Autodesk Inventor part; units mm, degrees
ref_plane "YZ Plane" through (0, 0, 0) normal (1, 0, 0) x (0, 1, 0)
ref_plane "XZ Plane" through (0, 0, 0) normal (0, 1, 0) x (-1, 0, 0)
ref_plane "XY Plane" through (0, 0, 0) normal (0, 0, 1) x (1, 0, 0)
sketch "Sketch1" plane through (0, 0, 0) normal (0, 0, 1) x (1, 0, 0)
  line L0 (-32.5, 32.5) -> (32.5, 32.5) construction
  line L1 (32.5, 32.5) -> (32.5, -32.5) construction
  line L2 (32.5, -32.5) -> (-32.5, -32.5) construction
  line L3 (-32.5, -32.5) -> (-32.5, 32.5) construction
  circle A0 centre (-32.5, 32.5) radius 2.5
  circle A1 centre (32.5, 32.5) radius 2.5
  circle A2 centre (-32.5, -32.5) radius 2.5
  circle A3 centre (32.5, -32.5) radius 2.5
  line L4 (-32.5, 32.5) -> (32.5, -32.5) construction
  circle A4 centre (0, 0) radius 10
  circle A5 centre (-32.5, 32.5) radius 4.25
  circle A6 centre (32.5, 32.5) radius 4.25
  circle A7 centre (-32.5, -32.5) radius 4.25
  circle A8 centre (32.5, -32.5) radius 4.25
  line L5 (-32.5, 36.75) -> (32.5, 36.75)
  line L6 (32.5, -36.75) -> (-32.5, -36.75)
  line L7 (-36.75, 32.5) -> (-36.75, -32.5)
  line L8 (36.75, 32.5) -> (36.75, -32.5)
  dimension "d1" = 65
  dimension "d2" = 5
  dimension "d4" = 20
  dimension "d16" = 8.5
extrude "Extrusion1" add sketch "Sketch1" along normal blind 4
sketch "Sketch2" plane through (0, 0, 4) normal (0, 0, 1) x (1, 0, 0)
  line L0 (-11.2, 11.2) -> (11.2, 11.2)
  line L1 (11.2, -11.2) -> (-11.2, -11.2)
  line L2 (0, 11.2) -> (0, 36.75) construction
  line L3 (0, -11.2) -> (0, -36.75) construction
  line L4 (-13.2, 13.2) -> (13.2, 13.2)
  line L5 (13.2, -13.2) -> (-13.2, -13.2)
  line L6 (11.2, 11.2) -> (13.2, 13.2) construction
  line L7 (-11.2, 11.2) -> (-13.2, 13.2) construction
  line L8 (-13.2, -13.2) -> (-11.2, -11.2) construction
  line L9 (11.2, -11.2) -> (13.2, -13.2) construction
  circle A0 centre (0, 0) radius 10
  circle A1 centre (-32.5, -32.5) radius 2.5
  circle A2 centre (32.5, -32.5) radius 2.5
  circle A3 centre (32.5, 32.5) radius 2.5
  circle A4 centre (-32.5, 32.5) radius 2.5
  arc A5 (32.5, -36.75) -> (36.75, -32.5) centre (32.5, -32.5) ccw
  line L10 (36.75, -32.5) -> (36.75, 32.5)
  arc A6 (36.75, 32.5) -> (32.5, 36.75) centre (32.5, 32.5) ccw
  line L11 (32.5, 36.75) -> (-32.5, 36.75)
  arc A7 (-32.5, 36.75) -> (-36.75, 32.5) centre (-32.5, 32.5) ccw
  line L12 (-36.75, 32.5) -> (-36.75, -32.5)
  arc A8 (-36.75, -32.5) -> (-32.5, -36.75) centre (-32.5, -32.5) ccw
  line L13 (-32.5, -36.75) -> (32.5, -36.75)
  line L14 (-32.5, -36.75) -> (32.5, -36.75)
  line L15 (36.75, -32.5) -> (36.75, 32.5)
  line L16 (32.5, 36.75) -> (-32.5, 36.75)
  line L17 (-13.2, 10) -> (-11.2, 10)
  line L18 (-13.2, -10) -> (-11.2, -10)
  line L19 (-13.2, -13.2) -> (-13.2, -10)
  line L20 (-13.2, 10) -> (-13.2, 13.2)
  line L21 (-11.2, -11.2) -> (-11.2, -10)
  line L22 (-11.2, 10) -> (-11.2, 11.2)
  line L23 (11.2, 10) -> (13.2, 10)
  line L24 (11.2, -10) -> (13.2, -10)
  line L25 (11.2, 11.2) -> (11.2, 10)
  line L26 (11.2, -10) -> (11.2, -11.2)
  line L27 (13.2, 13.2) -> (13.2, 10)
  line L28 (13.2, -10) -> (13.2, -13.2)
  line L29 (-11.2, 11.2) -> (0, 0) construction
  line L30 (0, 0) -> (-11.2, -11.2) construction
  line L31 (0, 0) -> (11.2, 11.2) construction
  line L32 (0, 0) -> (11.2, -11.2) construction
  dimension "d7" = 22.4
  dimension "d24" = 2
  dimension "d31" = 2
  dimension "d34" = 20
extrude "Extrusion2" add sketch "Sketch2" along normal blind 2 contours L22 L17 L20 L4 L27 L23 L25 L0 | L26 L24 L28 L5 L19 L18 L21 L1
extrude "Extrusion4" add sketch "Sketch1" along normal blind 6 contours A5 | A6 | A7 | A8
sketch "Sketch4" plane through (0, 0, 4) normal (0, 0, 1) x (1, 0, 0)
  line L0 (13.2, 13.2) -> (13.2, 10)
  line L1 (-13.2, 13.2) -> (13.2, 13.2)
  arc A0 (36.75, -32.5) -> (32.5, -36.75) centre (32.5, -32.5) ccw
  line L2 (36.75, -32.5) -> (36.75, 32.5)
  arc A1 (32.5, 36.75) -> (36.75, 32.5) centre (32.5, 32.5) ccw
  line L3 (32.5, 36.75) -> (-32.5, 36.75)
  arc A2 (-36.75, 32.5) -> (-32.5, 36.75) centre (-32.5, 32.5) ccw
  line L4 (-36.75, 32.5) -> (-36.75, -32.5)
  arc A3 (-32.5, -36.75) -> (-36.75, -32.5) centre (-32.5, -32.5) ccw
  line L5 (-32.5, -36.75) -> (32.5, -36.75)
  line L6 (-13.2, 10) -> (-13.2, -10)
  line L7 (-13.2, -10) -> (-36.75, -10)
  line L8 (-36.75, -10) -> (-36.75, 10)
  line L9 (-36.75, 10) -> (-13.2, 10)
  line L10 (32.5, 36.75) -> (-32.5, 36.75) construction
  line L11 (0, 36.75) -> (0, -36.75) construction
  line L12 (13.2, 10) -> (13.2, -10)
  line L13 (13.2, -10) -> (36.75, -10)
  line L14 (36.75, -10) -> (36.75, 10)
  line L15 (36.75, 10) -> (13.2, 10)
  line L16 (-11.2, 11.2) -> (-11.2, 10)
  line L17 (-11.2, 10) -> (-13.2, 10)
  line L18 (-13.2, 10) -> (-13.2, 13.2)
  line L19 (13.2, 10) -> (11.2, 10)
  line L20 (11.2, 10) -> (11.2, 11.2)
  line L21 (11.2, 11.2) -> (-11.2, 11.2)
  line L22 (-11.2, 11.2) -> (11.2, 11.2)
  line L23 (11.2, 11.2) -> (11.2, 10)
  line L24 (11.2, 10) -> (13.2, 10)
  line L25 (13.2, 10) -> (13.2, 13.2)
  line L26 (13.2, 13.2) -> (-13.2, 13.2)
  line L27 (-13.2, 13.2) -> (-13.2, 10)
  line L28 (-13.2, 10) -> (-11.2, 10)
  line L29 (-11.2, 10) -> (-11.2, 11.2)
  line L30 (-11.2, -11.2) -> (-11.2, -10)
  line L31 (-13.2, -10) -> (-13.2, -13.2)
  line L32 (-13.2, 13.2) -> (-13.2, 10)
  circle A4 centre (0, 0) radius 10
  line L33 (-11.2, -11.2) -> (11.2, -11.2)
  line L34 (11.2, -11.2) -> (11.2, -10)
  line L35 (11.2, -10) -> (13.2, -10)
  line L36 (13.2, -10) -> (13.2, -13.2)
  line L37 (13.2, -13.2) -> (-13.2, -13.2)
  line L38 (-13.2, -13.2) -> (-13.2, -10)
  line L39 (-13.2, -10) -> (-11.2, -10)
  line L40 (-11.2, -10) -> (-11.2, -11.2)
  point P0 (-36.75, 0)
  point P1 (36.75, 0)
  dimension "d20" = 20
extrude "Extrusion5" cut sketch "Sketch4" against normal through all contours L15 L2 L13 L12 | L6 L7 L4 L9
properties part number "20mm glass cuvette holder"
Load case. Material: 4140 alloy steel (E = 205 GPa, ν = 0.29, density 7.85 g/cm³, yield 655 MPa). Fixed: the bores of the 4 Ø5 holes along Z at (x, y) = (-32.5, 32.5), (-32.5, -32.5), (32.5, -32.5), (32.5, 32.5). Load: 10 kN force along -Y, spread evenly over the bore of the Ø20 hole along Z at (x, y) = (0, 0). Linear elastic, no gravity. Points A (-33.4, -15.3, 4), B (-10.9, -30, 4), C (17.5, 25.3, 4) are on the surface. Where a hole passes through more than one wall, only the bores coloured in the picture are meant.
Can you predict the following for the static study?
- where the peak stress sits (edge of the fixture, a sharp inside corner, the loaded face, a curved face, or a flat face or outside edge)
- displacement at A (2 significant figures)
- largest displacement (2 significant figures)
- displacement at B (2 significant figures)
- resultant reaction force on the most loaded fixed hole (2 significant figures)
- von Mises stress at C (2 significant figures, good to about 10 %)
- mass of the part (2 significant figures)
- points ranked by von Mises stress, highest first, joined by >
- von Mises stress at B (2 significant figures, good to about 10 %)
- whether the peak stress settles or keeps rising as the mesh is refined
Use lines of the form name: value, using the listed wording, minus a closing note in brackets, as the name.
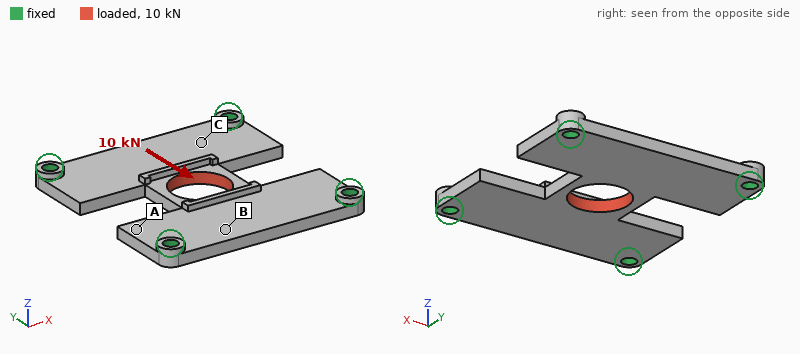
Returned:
where the peak stress sits: edge of the fixture
displacement at A: 4.1 µm
largest displacement: 17 µm
displacement at B: 13 µm
resultant reaction force on the most loaded fixed hole: 3.2 kN
von Mises stress at C: 58 MPa
mass of the part: 130 g
points ranked by von Mises stress, highest first, joined by >: C > B > A
von Mises stress at B: 31 MPa
whether the peak stress settles or keeps rising as the mesh is refined: keeps rising
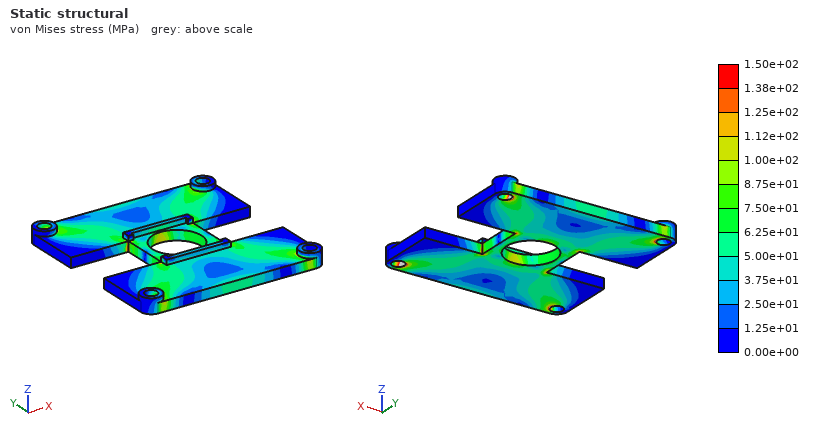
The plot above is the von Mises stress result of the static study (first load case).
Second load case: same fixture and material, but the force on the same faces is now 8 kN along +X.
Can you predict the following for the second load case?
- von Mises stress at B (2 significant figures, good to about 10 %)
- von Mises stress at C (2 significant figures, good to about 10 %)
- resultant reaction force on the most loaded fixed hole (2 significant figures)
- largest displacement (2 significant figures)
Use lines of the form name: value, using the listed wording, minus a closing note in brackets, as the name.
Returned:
von Mises stress at B: 14 MPa
von Mises stress at C: 29 MPa
resultant reaction force on the most loaded fixed hole: 2.4 kN
largest displacement: 19 µm
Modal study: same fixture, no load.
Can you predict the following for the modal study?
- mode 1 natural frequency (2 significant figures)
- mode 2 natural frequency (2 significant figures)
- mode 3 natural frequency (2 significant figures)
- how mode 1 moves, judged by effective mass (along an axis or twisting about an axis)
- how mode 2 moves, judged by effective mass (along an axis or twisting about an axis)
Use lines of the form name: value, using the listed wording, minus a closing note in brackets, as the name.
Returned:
mode 1 natural frequency: 3400 Hz
mode 2 natural frequency: 5300 Hz
mode 3 natural frequency: 6900 Hz
how mode 1 moves, judged by effective mass: along Z
how mode 2 moves, judged by effective mass: twisting about X
